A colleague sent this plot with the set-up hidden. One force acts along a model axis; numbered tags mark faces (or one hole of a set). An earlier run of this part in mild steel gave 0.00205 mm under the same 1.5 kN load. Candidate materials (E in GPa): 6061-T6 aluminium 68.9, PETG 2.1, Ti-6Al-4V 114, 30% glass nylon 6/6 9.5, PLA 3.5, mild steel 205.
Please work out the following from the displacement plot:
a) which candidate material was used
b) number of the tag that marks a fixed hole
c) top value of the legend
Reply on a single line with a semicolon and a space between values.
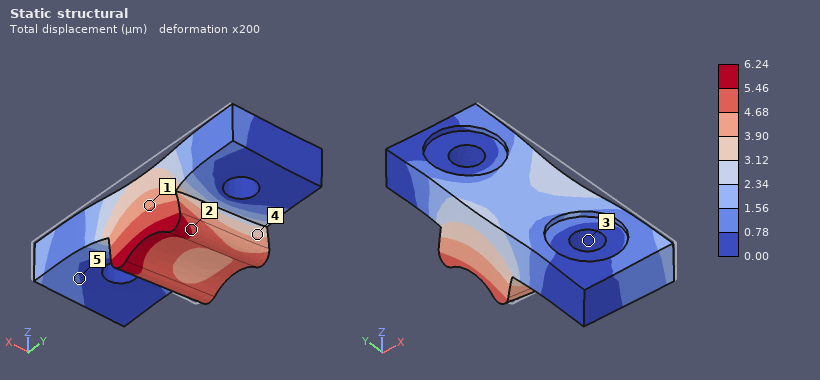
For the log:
6061-T6 aluminium; 3; 6.24 µm
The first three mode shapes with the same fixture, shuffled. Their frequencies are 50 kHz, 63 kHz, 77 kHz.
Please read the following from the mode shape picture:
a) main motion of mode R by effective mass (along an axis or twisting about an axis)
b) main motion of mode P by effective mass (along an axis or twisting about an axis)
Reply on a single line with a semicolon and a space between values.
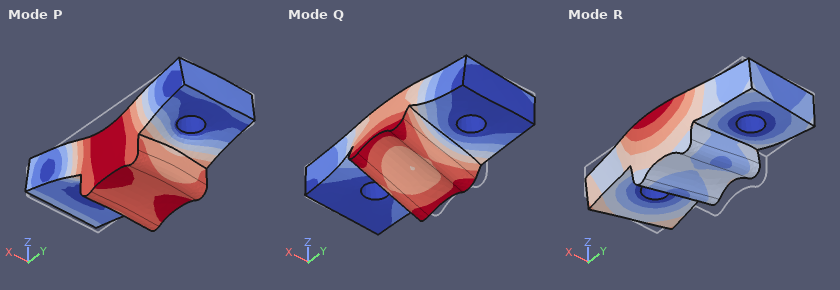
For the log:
along X; along Z
